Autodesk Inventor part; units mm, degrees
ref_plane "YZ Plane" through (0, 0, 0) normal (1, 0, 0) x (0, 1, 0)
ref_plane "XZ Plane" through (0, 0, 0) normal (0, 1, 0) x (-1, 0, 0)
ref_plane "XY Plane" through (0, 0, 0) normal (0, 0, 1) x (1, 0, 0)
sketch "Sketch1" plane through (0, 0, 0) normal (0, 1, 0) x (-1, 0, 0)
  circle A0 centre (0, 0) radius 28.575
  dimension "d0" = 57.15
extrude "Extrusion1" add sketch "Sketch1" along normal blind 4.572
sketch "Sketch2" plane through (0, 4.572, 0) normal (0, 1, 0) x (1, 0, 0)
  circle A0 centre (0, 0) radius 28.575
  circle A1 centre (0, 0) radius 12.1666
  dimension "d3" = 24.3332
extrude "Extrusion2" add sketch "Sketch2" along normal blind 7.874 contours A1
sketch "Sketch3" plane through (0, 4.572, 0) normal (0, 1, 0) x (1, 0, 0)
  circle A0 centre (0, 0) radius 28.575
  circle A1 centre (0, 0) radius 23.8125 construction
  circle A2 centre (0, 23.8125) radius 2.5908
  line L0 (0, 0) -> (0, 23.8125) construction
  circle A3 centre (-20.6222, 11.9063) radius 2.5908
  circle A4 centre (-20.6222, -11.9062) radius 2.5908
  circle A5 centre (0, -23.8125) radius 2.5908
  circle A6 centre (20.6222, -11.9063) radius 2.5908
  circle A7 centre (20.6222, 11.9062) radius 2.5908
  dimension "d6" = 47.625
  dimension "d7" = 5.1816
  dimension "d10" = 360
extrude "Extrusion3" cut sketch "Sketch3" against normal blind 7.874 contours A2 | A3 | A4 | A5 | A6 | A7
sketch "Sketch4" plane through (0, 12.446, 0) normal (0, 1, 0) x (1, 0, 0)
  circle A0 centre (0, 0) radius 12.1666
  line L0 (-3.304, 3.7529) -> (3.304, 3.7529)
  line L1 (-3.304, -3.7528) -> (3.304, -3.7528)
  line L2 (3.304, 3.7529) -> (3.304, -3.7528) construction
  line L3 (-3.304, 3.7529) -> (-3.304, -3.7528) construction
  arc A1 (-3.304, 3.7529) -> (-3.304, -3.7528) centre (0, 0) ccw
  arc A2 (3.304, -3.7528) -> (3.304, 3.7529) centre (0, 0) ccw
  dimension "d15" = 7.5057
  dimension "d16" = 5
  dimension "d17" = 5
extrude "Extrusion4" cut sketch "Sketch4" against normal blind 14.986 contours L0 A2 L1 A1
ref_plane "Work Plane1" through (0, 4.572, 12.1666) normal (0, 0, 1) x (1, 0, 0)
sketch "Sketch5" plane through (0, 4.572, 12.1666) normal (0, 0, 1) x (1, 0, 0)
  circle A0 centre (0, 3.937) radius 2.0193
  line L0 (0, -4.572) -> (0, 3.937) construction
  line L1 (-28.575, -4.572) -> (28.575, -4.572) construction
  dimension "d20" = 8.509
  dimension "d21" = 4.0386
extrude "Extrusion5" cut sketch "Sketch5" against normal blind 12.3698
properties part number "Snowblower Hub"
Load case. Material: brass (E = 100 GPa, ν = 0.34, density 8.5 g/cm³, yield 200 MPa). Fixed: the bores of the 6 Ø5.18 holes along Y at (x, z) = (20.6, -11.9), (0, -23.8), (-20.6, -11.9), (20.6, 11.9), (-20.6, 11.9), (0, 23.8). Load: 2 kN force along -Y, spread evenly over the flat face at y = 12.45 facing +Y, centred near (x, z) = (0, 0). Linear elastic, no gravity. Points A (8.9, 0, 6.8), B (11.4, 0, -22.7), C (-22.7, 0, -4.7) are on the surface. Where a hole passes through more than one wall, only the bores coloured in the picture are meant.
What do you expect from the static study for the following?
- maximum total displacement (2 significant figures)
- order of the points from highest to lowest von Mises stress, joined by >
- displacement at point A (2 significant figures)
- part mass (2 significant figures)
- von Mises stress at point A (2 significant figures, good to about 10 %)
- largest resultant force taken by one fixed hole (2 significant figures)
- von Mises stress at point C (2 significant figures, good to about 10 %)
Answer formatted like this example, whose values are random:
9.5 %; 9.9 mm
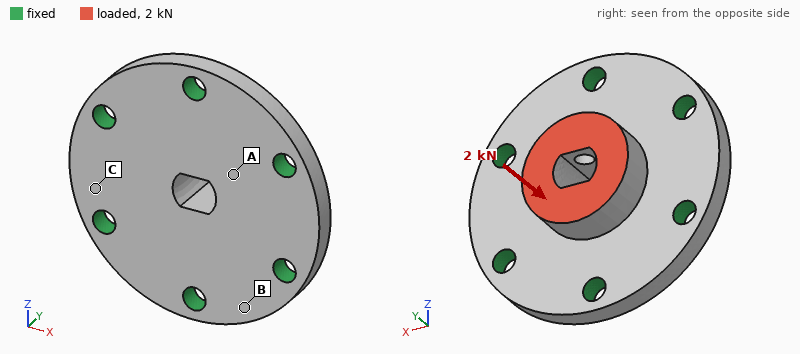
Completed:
7.9 µm; A > C > B; 6.4 µm; 120 g; 18 MPa; 370 N; 9.7 MPa
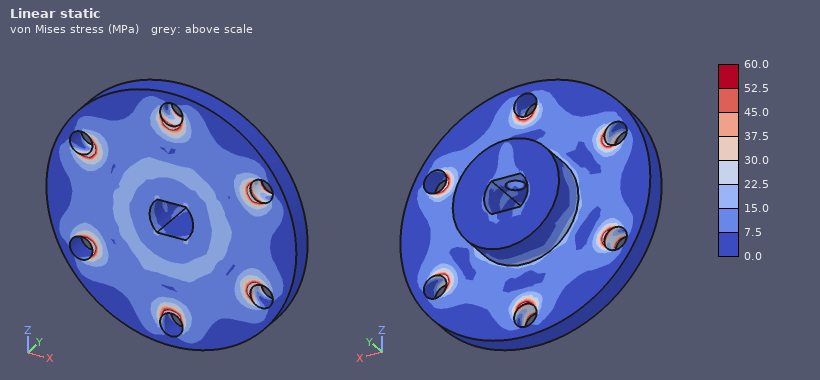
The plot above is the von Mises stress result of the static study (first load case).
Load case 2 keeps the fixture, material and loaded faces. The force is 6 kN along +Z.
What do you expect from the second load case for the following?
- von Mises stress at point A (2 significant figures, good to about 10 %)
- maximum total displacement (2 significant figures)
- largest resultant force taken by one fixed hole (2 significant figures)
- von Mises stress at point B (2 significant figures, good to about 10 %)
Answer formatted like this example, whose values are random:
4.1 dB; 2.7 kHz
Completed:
39 MPa; 28 µm; 1.9 kN; 16 MPa
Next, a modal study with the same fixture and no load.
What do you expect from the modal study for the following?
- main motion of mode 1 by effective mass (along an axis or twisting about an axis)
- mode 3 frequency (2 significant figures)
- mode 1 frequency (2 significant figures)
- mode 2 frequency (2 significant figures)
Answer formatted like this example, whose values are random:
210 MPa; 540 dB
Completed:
along Y; 17 kHz; 12 kHz; 17 kHz
